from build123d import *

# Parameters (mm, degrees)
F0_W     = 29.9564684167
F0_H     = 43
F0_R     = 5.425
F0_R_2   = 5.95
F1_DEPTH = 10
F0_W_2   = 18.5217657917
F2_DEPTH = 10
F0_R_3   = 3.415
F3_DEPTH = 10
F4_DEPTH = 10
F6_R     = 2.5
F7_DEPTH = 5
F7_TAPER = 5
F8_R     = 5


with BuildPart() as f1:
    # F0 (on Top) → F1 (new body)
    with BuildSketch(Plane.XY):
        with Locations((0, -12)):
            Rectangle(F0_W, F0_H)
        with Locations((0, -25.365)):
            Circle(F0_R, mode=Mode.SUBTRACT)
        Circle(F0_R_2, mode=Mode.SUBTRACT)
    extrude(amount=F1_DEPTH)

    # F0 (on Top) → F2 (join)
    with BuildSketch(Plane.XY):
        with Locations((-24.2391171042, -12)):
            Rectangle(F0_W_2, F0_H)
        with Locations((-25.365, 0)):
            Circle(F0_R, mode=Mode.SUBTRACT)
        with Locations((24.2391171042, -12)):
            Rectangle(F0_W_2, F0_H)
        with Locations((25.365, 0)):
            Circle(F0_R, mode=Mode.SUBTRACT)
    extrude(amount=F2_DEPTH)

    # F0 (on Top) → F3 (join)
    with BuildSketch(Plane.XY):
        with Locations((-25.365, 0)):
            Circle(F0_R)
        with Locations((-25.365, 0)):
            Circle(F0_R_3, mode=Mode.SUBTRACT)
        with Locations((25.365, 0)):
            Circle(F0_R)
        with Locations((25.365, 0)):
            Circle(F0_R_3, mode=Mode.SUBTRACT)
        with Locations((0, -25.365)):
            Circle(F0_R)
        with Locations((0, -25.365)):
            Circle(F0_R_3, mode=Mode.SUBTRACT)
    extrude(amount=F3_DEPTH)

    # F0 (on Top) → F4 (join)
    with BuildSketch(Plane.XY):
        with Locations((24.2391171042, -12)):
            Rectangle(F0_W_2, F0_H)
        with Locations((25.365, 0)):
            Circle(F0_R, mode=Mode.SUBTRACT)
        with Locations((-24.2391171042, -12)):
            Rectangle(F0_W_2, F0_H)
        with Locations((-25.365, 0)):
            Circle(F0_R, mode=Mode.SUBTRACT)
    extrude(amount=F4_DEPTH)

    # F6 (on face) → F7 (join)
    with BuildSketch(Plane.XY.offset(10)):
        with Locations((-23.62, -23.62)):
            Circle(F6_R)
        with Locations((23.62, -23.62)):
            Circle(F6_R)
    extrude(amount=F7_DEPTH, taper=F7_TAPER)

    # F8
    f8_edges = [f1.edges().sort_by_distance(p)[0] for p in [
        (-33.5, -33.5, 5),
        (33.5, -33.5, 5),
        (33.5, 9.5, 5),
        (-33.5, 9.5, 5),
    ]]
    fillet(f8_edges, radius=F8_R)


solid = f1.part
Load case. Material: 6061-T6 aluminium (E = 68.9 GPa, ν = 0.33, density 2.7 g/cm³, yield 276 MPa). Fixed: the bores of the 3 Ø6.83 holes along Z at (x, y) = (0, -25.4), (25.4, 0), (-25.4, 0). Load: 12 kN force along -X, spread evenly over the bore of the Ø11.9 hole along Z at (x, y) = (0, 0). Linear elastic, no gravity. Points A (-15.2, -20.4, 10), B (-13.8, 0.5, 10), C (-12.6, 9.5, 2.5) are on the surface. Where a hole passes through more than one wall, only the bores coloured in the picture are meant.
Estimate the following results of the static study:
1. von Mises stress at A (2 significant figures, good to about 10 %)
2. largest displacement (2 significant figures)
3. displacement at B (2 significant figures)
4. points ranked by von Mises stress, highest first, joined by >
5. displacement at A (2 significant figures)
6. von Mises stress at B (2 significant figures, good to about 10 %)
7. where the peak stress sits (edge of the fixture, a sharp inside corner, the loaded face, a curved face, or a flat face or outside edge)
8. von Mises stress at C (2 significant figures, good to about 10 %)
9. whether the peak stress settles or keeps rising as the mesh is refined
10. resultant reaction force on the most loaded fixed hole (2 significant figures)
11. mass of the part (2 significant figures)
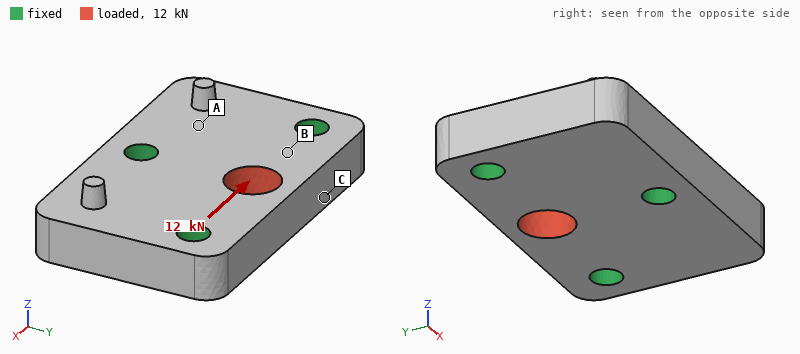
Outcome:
5.9 MPa
12 µm
4.6 µm
B > C > A
2.2 µm
36 MPa
edge of the fixture
27 MPa
keeps rising
5.0 kN
72 g
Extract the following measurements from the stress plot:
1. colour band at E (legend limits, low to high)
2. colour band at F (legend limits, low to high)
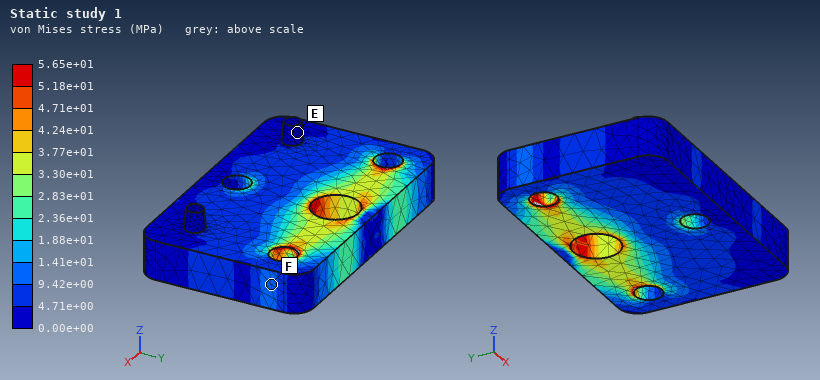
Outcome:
0.00e+00 to 4.71e+00 MPa
9.42e+00 to 1.41e+01 MPa
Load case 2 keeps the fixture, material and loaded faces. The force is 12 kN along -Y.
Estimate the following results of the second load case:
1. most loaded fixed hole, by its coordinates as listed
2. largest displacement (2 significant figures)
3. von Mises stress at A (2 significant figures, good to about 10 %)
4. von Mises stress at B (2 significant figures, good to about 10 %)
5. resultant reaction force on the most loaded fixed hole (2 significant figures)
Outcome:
(0, -25.4)
31 µm
11 MPa
24 MPa
6.4 kN
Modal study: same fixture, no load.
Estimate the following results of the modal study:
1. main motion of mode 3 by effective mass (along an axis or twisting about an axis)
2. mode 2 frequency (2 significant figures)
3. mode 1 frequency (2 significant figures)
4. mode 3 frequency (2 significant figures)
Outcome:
along Z
13 kHz
13 kHz
21 kHz
